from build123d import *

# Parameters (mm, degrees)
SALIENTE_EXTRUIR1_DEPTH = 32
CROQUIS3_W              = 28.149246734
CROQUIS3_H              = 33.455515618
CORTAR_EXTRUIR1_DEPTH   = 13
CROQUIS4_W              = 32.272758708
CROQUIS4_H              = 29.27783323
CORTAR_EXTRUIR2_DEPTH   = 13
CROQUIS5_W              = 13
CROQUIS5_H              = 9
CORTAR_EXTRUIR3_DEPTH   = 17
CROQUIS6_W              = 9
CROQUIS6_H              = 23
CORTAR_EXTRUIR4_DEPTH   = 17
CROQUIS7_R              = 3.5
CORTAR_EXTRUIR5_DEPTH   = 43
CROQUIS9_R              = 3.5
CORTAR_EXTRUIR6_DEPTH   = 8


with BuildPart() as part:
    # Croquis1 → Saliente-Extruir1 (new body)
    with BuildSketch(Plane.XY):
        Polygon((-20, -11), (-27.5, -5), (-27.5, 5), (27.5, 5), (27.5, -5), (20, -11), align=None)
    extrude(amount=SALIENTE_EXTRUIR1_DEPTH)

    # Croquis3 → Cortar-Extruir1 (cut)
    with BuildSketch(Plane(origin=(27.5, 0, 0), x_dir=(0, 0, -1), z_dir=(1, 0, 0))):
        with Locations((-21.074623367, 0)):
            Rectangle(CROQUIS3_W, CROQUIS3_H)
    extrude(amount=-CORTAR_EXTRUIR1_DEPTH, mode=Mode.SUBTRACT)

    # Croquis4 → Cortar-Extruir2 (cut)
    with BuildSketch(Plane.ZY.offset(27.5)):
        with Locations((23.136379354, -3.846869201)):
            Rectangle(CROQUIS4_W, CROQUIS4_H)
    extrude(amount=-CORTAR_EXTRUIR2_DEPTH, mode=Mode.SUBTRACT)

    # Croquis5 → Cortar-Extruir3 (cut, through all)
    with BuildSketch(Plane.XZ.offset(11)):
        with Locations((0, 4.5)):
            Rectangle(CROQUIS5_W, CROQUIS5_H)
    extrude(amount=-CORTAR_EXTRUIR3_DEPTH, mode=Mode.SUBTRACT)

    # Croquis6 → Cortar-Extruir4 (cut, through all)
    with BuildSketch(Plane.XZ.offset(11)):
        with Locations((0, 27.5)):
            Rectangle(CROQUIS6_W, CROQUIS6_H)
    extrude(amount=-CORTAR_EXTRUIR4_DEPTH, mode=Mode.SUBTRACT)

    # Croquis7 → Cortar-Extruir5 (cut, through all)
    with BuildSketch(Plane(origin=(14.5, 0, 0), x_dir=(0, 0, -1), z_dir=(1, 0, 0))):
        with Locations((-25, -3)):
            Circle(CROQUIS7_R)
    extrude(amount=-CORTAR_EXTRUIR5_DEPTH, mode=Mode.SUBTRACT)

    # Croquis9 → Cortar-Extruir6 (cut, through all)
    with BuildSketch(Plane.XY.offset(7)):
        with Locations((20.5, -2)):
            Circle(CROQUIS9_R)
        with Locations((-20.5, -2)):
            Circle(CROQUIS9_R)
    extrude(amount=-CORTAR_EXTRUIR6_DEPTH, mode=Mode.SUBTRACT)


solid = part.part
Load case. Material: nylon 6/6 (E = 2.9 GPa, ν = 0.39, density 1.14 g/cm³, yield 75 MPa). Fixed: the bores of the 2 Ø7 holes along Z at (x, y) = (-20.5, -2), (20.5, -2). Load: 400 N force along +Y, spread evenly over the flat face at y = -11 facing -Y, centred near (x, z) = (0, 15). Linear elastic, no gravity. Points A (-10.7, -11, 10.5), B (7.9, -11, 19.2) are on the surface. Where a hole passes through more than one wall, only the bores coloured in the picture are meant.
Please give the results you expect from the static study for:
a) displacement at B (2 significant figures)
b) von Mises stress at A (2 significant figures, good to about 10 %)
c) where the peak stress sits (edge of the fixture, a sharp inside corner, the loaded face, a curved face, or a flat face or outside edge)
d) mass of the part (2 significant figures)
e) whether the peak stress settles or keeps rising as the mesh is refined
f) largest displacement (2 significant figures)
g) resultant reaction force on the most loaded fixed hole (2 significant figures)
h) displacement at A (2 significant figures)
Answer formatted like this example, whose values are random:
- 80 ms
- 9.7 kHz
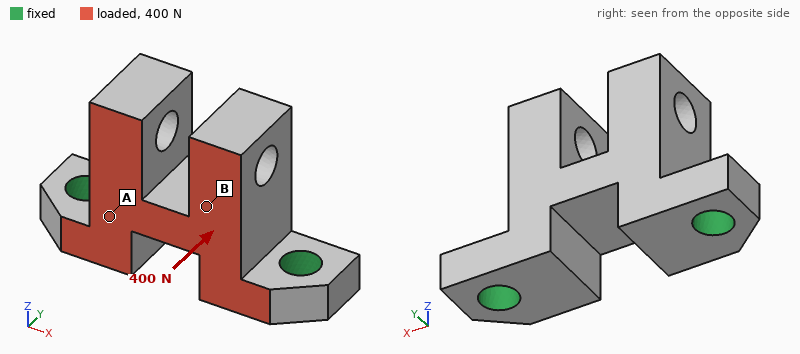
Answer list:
- 0.19 mm
- 3.9 MPa
- edge of the fixture
- 14 g
- keeps rising
- 0.32 mm
- 200 N
- 0.11 mm
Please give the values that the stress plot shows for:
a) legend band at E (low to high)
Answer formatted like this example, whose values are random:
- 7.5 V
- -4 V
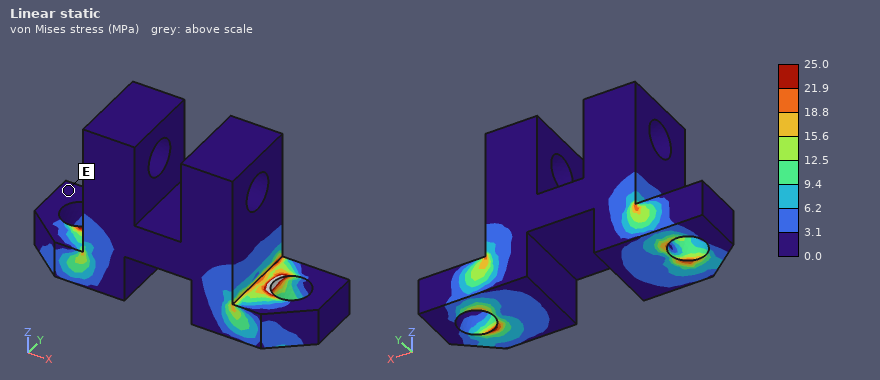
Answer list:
- 0.0 to 3.1 MPa
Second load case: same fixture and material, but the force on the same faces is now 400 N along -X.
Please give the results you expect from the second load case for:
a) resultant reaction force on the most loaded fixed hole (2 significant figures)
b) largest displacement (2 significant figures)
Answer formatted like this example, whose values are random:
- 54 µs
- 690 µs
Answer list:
- 250 N
- 0.12 mm
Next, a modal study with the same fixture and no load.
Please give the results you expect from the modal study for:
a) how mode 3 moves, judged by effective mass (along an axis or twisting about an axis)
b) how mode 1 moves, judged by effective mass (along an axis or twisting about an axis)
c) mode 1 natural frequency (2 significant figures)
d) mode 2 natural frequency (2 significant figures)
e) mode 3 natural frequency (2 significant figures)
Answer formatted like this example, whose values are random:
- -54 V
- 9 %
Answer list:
- along X
- along Y
- 2000 Hz
- 3500 Hz
- 4100 Hz
